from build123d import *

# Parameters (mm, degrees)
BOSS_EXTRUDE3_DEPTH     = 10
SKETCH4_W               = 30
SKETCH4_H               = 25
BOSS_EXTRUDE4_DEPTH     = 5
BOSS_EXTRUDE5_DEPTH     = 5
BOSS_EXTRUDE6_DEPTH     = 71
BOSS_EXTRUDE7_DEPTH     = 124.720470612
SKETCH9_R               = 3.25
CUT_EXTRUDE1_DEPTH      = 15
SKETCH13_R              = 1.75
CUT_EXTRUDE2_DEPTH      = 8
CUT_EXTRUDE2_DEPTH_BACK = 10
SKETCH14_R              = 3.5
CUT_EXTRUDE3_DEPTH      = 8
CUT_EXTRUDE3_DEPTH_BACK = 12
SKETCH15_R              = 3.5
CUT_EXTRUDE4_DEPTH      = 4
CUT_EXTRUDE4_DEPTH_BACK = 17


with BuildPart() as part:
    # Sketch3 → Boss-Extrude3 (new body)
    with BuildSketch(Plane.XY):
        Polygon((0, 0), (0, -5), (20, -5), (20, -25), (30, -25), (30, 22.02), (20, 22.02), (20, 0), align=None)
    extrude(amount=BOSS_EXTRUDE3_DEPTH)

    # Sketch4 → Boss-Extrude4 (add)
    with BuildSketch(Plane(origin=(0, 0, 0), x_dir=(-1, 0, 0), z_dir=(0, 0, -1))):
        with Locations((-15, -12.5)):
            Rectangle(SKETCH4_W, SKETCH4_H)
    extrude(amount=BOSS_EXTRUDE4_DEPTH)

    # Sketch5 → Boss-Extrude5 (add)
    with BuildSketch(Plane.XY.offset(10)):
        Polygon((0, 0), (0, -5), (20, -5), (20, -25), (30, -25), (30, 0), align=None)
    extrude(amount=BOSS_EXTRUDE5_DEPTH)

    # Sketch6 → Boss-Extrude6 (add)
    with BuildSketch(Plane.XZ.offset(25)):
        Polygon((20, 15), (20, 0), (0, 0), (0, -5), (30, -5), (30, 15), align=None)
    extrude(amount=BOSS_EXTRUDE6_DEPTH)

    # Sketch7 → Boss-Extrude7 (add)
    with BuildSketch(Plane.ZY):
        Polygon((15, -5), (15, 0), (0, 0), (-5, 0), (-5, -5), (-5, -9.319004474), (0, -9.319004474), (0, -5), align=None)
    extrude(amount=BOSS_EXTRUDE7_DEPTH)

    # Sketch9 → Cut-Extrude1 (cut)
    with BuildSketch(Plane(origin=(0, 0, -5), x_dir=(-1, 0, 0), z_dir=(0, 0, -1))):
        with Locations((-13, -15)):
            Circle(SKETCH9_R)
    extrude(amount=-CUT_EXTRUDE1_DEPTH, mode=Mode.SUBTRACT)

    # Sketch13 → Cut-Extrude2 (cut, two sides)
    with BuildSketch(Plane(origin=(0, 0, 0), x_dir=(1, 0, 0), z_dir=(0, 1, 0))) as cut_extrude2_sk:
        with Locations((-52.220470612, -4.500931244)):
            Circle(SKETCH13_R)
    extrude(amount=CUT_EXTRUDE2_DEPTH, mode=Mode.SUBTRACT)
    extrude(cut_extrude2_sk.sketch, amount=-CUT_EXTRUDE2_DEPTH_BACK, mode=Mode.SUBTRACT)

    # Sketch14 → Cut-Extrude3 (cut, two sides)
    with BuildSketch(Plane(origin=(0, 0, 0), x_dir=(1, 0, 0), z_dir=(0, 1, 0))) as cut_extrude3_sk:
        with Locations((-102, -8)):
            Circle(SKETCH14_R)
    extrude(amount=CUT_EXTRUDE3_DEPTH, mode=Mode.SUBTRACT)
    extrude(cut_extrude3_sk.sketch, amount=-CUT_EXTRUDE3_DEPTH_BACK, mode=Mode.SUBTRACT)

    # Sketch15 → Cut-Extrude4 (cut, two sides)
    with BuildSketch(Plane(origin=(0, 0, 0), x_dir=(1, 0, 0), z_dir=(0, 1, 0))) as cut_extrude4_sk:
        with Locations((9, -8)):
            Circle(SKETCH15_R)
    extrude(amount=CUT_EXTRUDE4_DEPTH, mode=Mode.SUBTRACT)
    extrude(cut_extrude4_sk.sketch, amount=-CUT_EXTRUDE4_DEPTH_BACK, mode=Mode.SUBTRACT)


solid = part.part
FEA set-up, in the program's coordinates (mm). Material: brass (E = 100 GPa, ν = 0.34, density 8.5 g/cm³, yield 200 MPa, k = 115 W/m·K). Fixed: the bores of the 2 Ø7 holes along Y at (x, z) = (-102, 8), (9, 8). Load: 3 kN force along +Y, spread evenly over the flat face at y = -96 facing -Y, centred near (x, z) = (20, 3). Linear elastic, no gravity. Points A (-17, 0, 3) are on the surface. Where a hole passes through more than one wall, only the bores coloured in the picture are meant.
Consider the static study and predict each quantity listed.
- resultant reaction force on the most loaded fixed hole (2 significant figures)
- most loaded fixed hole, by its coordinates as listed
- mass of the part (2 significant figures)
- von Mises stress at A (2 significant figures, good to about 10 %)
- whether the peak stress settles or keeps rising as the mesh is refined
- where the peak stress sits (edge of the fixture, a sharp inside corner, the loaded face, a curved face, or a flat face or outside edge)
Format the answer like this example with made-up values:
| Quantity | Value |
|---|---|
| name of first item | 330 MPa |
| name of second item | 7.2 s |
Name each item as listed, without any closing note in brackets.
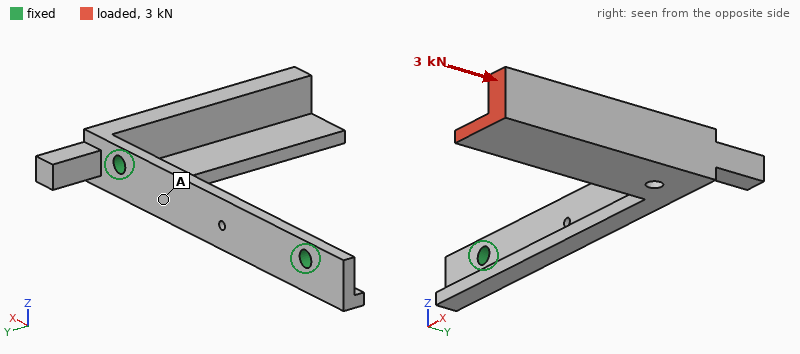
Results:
| Quantity | Value |
|---|---|
| resultant reaction force on the most loaded fixed hole | 3.1 kN |
| most loaded fixed hole, by its coordinates as listed | (9, 8) |
| mass of the part | 400 g |
| von Mises stress at A | 16 MPa |
| whether the peak stress settles or keeps rising as the mesh is refined | keeps rising |
| where the peak stress sits | edge of the fixture |
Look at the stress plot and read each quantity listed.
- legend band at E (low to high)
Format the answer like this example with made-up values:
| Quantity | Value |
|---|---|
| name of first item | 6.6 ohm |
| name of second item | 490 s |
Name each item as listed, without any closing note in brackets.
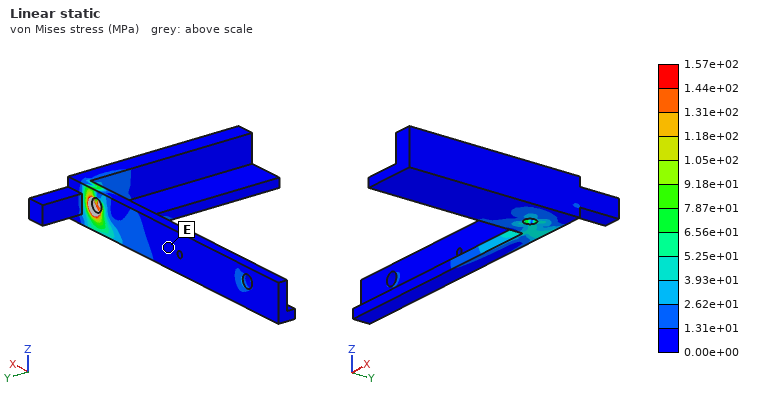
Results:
| Quantity | Value |
|---|---|
| legend band at E | 0.00e+00 to 1.31e+01 MPa |
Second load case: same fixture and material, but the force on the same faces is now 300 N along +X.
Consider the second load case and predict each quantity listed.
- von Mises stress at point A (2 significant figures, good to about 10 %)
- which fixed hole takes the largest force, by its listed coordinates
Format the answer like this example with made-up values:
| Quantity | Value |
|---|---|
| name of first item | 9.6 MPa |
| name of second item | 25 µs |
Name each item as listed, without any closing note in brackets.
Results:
| Quantity | Value |
|---|---|
| von Mises stress at point A | 20 MPa |
| which fixed hole takes the largest force, by its listed coordinates | (-102, 8) |
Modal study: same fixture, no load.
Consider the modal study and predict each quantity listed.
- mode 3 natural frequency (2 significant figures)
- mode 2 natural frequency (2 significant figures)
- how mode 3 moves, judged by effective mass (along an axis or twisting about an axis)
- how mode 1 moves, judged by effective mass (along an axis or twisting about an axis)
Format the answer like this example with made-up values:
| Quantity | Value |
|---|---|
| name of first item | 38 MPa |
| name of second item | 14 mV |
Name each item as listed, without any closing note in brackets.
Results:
| Quantity | Value |
|---|---|
| mode 3 natural frequency | 2000 Hz |
| mode 2 natural frequency | 580 Hz |
| how mode 3 moves, judged by effective mass | along Y |
| how mode 1 moves, judged by effective mass | along Z |
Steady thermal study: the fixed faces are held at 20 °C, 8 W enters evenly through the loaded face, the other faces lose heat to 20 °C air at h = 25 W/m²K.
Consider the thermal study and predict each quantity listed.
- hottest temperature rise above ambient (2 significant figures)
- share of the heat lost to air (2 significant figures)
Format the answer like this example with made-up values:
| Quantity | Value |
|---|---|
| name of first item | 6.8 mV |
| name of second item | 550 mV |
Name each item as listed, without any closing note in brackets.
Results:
| Quantity | Value |
|---|---|
| hottest temperature rise above ambient | 21 K |
| share of the heat lost to air | 35 % |
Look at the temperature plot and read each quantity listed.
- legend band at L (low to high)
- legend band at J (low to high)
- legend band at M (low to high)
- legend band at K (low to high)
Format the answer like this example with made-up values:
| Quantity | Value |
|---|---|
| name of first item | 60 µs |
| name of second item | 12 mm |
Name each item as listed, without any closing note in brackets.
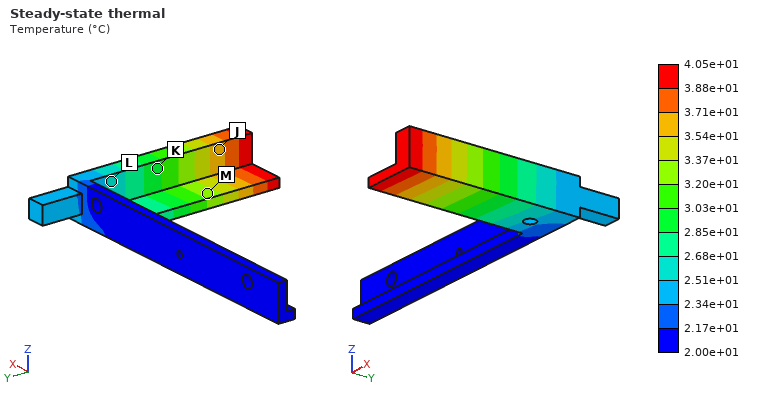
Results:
| Quantity | Value |
|---|---|
| legend band at L | 2.51e+01 to 2.68e+01 °C |
| legend band at J | 3.54e+01 to 3.71e+01 °C |
| legend band at M | 3.20e+01 to 3.37e+01 °C |
| legend band at K | 2.85e+01 to 3.03e+01 °C |
